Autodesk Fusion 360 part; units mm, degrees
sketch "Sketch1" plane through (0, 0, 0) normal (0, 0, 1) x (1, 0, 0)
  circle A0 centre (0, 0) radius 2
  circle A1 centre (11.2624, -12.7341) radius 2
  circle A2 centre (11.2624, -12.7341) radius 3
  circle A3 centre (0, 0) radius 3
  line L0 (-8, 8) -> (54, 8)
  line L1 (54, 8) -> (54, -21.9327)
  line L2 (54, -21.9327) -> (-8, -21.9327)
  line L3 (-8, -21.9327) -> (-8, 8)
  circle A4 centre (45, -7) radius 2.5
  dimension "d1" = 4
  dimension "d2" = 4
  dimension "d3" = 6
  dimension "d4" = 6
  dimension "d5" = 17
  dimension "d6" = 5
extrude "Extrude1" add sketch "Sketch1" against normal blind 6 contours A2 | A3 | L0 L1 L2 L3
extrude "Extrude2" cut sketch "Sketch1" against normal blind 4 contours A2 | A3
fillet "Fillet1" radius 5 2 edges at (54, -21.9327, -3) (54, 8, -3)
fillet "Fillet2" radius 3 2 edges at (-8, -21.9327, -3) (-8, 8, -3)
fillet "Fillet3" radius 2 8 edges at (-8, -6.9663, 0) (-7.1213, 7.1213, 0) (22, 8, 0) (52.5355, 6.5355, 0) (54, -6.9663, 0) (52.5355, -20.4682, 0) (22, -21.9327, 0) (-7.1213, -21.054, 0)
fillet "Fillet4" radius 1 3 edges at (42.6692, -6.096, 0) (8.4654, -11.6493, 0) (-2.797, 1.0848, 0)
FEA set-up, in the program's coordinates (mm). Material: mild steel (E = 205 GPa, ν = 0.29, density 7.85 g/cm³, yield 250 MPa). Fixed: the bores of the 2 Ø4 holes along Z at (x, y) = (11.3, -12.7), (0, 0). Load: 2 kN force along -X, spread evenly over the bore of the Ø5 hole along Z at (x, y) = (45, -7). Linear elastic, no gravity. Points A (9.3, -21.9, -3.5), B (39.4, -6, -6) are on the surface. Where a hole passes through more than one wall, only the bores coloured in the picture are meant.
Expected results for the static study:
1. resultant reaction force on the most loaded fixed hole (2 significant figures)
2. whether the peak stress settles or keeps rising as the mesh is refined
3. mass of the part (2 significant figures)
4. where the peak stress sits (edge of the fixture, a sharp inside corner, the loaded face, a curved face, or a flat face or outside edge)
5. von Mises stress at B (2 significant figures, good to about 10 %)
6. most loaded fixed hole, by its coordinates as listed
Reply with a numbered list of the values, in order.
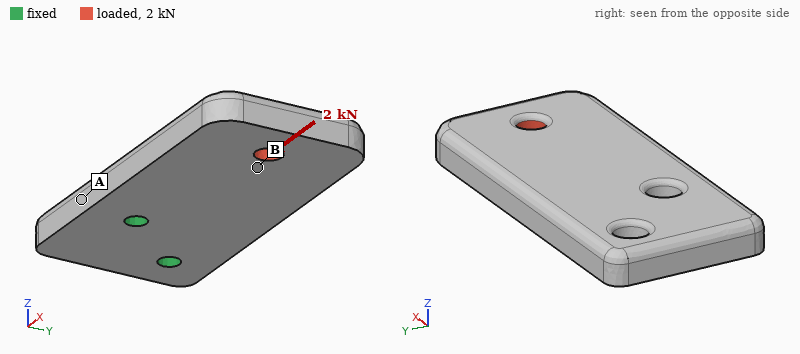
1. 1.1 kN
2. keeps rising
3. 82 g
4. edge of the fixture
5. 27 MPa
6. (11.3, -12.7)
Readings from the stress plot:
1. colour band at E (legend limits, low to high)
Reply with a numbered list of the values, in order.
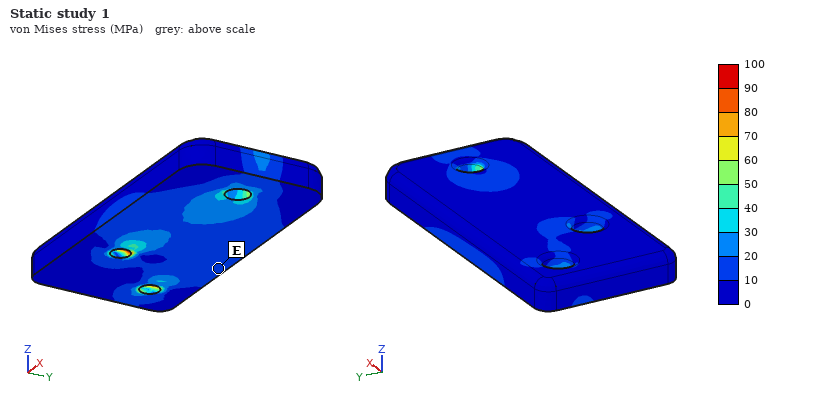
1. 10 to 20 MPa
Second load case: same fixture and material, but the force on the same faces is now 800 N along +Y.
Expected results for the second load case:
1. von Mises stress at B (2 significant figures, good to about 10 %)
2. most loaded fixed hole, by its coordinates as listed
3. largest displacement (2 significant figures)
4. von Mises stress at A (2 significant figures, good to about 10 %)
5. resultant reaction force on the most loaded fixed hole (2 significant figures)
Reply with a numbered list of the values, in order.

1. 16 MPa
2. (11.3, -12.7)
3. 21 µm
4. 25 MPa
5. 1.9 kN
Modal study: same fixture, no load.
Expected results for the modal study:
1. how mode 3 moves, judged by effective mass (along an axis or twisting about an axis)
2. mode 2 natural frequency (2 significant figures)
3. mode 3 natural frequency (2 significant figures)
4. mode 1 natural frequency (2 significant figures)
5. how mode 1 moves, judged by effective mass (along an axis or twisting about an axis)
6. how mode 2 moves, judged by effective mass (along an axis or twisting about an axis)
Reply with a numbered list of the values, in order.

1. along Y
2. 5900 Hz
3. 6700 Hz
4. 1800 Hz
5. along Z
6. twisting about X
